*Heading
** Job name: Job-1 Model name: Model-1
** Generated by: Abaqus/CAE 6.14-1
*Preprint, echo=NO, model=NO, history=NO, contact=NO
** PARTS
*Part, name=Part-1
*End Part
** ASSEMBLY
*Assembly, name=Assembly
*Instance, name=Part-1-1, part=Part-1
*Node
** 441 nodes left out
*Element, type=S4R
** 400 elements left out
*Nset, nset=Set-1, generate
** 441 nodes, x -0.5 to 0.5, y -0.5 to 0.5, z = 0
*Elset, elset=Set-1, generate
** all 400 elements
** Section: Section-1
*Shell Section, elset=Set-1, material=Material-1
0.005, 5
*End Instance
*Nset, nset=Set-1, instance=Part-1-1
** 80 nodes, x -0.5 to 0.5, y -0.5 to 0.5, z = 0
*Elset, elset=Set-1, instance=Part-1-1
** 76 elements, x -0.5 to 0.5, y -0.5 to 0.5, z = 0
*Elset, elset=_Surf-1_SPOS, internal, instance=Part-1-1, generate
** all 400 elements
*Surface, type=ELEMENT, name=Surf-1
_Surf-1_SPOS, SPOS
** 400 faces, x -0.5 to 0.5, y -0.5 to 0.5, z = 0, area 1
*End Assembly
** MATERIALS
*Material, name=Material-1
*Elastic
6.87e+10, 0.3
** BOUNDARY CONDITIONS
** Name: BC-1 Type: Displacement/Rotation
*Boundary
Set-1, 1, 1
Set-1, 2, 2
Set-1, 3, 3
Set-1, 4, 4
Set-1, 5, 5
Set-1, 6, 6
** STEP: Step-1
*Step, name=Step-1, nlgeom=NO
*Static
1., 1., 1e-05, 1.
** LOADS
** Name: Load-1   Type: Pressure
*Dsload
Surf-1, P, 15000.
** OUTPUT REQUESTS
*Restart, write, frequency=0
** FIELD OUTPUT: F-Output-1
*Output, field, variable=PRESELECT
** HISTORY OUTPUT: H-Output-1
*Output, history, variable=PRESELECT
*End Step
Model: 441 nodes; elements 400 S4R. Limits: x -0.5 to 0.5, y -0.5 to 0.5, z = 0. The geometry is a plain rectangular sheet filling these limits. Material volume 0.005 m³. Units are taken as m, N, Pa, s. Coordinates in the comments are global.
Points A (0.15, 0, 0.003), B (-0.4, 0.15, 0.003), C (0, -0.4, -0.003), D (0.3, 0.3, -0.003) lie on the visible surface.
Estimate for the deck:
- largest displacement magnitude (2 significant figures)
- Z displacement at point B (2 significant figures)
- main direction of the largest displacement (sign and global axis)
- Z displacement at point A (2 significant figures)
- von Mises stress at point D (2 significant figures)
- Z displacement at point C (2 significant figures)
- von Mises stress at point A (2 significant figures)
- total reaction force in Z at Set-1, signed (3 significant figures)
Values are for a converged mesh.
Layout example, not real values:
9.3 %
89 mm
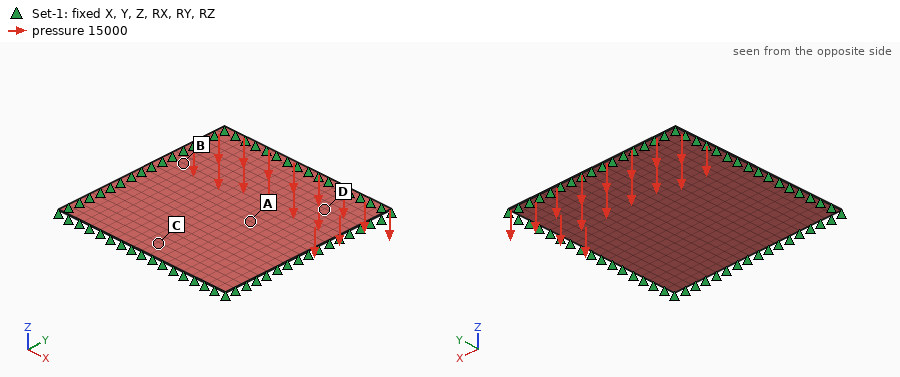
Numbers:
0.024 m
-0.0030 m
-Z
-0.020 m
5.3e+07 Pa
-0.0036 m
6.9e+07 Pa
15000 N
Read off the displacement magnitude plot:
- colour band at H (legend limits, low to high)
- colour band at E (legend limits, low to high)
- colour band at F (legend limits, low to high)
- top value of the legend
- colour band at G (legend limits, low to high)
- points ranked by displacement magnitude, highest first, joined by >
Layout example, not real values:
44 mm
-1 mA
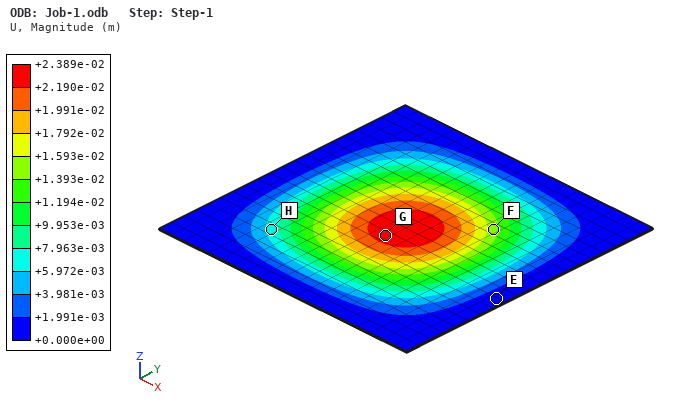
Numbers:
+5.972e-03 to +7.963e-03 m
+0.000e+00 to +1.991e-03 m
+1.393e-02 to +1.593e-02 m
+2.389e-02 m
+2.190e-02 to +2.389e-02 m
G > F > H > E
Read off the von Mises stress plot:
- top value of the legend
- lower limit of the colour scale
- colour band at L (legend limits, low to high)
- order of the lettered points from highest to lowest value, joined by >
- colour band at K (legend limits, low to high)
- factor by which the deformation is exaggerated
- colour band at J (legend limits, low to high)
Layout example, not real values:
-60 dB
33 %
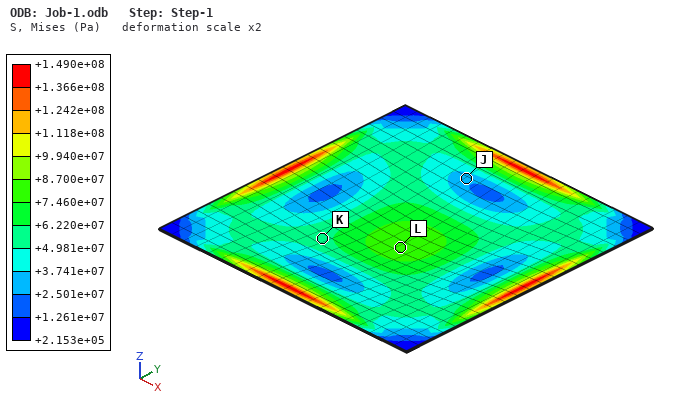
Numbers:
+1.490e+08 Pa
+2.153e+05 Pa
+7.460e+07 to +8.700e+07 Pa
L > K > J
+4.981e+07 to +6.220e+07 Pa
2
+2.501e+07 to +3.741e+07 Pa
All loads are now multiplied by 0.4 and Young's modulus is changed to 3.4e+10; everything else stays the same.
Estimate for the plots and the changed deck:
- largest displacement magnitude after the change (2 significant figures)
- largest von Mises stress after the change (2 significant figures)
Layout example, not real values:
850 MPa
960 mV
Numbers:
0.019 m
6.0e+07 Pa
